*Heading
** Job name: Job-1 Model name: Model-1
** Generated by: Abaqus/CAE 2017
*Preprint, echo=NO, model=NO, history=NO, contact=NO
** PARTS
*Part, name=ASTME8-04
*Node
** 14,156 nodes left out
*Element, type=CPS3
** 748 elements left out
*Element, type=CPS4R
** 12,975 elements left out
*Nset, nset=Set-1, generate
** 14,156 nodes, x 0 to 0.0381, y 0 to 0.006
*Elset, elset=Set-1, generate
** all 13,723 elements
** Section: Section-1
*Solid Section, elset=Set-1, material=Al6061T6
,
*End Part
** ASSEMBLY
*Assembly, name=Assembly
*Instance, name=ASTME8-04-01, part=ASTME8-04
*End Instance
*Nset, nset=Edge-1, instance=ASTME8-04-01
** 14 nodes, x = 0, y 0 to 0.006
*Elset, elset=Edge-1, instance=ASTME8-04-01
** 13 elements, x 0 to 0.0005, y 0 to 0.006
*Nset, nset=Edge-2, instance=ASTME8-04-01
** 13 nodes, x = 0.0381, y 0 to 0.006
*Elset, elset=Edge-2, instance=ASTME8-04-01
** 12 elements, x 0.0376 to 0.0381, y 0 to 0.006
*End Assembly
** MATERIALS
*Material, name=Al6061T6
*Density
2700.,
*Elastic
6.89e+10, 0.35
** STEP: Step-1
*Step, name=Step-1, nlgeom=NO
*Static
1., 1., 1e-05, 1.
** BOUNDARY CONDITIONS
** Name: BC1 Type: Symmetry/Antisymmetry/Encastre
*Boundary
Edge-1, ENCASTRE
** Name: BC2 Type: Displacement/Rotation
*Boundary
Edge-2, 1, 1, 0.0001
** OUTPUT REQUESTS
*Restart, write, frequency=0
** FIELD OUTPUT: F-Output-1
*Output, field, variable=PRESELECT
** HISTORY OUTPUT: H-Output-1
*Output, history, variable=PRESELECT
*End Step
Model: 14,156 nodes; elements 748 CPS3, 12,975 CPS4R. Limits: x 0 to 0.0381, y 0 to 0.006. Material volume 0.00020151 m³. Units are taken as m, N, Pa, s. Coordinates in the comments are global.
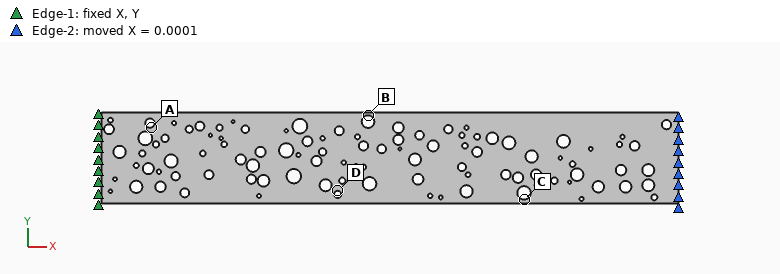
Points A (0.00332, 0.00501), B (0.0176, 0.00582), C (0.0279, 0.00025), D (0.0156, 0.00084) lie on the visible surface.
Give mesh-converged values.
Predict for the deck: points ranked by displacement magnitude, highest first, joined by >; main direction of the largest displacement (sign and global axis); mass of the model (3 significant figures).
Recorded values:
C > B > D > A
+X
0.544 kg
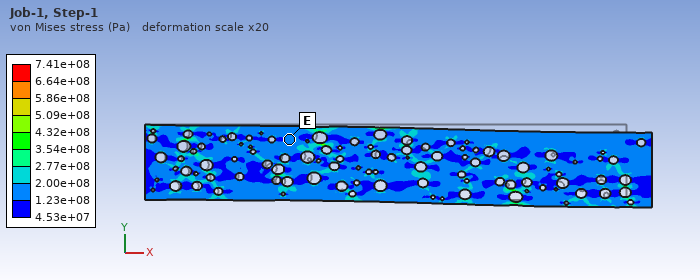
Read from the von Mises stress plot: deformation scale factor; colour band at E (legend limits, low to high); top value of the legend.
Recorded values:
20
1.23e+08 to 2.00e+08 Pa
7.41e+08 Pa
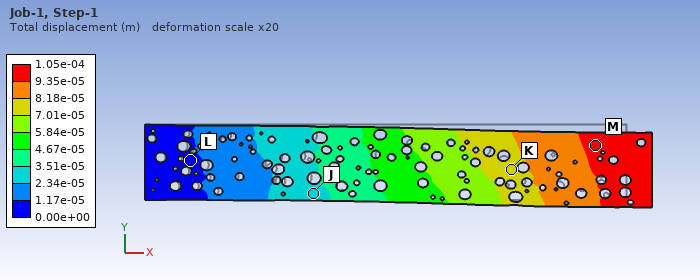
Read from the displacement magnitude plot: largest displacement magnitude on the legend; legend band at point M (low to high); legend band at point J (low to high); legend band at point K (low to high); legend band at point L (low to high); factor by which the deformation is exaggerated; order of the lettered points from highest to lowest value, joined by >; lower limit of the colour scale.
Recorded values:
1.05e-04 m
9.35e-05 to 1.05e-04 m
2.34e-05 to 3.51e-05 m
7.01e-05 to 8.18e-05 m
0.00e+00 to 1.17e-05 m
20
M > K > J > L
0.00e+00 m
